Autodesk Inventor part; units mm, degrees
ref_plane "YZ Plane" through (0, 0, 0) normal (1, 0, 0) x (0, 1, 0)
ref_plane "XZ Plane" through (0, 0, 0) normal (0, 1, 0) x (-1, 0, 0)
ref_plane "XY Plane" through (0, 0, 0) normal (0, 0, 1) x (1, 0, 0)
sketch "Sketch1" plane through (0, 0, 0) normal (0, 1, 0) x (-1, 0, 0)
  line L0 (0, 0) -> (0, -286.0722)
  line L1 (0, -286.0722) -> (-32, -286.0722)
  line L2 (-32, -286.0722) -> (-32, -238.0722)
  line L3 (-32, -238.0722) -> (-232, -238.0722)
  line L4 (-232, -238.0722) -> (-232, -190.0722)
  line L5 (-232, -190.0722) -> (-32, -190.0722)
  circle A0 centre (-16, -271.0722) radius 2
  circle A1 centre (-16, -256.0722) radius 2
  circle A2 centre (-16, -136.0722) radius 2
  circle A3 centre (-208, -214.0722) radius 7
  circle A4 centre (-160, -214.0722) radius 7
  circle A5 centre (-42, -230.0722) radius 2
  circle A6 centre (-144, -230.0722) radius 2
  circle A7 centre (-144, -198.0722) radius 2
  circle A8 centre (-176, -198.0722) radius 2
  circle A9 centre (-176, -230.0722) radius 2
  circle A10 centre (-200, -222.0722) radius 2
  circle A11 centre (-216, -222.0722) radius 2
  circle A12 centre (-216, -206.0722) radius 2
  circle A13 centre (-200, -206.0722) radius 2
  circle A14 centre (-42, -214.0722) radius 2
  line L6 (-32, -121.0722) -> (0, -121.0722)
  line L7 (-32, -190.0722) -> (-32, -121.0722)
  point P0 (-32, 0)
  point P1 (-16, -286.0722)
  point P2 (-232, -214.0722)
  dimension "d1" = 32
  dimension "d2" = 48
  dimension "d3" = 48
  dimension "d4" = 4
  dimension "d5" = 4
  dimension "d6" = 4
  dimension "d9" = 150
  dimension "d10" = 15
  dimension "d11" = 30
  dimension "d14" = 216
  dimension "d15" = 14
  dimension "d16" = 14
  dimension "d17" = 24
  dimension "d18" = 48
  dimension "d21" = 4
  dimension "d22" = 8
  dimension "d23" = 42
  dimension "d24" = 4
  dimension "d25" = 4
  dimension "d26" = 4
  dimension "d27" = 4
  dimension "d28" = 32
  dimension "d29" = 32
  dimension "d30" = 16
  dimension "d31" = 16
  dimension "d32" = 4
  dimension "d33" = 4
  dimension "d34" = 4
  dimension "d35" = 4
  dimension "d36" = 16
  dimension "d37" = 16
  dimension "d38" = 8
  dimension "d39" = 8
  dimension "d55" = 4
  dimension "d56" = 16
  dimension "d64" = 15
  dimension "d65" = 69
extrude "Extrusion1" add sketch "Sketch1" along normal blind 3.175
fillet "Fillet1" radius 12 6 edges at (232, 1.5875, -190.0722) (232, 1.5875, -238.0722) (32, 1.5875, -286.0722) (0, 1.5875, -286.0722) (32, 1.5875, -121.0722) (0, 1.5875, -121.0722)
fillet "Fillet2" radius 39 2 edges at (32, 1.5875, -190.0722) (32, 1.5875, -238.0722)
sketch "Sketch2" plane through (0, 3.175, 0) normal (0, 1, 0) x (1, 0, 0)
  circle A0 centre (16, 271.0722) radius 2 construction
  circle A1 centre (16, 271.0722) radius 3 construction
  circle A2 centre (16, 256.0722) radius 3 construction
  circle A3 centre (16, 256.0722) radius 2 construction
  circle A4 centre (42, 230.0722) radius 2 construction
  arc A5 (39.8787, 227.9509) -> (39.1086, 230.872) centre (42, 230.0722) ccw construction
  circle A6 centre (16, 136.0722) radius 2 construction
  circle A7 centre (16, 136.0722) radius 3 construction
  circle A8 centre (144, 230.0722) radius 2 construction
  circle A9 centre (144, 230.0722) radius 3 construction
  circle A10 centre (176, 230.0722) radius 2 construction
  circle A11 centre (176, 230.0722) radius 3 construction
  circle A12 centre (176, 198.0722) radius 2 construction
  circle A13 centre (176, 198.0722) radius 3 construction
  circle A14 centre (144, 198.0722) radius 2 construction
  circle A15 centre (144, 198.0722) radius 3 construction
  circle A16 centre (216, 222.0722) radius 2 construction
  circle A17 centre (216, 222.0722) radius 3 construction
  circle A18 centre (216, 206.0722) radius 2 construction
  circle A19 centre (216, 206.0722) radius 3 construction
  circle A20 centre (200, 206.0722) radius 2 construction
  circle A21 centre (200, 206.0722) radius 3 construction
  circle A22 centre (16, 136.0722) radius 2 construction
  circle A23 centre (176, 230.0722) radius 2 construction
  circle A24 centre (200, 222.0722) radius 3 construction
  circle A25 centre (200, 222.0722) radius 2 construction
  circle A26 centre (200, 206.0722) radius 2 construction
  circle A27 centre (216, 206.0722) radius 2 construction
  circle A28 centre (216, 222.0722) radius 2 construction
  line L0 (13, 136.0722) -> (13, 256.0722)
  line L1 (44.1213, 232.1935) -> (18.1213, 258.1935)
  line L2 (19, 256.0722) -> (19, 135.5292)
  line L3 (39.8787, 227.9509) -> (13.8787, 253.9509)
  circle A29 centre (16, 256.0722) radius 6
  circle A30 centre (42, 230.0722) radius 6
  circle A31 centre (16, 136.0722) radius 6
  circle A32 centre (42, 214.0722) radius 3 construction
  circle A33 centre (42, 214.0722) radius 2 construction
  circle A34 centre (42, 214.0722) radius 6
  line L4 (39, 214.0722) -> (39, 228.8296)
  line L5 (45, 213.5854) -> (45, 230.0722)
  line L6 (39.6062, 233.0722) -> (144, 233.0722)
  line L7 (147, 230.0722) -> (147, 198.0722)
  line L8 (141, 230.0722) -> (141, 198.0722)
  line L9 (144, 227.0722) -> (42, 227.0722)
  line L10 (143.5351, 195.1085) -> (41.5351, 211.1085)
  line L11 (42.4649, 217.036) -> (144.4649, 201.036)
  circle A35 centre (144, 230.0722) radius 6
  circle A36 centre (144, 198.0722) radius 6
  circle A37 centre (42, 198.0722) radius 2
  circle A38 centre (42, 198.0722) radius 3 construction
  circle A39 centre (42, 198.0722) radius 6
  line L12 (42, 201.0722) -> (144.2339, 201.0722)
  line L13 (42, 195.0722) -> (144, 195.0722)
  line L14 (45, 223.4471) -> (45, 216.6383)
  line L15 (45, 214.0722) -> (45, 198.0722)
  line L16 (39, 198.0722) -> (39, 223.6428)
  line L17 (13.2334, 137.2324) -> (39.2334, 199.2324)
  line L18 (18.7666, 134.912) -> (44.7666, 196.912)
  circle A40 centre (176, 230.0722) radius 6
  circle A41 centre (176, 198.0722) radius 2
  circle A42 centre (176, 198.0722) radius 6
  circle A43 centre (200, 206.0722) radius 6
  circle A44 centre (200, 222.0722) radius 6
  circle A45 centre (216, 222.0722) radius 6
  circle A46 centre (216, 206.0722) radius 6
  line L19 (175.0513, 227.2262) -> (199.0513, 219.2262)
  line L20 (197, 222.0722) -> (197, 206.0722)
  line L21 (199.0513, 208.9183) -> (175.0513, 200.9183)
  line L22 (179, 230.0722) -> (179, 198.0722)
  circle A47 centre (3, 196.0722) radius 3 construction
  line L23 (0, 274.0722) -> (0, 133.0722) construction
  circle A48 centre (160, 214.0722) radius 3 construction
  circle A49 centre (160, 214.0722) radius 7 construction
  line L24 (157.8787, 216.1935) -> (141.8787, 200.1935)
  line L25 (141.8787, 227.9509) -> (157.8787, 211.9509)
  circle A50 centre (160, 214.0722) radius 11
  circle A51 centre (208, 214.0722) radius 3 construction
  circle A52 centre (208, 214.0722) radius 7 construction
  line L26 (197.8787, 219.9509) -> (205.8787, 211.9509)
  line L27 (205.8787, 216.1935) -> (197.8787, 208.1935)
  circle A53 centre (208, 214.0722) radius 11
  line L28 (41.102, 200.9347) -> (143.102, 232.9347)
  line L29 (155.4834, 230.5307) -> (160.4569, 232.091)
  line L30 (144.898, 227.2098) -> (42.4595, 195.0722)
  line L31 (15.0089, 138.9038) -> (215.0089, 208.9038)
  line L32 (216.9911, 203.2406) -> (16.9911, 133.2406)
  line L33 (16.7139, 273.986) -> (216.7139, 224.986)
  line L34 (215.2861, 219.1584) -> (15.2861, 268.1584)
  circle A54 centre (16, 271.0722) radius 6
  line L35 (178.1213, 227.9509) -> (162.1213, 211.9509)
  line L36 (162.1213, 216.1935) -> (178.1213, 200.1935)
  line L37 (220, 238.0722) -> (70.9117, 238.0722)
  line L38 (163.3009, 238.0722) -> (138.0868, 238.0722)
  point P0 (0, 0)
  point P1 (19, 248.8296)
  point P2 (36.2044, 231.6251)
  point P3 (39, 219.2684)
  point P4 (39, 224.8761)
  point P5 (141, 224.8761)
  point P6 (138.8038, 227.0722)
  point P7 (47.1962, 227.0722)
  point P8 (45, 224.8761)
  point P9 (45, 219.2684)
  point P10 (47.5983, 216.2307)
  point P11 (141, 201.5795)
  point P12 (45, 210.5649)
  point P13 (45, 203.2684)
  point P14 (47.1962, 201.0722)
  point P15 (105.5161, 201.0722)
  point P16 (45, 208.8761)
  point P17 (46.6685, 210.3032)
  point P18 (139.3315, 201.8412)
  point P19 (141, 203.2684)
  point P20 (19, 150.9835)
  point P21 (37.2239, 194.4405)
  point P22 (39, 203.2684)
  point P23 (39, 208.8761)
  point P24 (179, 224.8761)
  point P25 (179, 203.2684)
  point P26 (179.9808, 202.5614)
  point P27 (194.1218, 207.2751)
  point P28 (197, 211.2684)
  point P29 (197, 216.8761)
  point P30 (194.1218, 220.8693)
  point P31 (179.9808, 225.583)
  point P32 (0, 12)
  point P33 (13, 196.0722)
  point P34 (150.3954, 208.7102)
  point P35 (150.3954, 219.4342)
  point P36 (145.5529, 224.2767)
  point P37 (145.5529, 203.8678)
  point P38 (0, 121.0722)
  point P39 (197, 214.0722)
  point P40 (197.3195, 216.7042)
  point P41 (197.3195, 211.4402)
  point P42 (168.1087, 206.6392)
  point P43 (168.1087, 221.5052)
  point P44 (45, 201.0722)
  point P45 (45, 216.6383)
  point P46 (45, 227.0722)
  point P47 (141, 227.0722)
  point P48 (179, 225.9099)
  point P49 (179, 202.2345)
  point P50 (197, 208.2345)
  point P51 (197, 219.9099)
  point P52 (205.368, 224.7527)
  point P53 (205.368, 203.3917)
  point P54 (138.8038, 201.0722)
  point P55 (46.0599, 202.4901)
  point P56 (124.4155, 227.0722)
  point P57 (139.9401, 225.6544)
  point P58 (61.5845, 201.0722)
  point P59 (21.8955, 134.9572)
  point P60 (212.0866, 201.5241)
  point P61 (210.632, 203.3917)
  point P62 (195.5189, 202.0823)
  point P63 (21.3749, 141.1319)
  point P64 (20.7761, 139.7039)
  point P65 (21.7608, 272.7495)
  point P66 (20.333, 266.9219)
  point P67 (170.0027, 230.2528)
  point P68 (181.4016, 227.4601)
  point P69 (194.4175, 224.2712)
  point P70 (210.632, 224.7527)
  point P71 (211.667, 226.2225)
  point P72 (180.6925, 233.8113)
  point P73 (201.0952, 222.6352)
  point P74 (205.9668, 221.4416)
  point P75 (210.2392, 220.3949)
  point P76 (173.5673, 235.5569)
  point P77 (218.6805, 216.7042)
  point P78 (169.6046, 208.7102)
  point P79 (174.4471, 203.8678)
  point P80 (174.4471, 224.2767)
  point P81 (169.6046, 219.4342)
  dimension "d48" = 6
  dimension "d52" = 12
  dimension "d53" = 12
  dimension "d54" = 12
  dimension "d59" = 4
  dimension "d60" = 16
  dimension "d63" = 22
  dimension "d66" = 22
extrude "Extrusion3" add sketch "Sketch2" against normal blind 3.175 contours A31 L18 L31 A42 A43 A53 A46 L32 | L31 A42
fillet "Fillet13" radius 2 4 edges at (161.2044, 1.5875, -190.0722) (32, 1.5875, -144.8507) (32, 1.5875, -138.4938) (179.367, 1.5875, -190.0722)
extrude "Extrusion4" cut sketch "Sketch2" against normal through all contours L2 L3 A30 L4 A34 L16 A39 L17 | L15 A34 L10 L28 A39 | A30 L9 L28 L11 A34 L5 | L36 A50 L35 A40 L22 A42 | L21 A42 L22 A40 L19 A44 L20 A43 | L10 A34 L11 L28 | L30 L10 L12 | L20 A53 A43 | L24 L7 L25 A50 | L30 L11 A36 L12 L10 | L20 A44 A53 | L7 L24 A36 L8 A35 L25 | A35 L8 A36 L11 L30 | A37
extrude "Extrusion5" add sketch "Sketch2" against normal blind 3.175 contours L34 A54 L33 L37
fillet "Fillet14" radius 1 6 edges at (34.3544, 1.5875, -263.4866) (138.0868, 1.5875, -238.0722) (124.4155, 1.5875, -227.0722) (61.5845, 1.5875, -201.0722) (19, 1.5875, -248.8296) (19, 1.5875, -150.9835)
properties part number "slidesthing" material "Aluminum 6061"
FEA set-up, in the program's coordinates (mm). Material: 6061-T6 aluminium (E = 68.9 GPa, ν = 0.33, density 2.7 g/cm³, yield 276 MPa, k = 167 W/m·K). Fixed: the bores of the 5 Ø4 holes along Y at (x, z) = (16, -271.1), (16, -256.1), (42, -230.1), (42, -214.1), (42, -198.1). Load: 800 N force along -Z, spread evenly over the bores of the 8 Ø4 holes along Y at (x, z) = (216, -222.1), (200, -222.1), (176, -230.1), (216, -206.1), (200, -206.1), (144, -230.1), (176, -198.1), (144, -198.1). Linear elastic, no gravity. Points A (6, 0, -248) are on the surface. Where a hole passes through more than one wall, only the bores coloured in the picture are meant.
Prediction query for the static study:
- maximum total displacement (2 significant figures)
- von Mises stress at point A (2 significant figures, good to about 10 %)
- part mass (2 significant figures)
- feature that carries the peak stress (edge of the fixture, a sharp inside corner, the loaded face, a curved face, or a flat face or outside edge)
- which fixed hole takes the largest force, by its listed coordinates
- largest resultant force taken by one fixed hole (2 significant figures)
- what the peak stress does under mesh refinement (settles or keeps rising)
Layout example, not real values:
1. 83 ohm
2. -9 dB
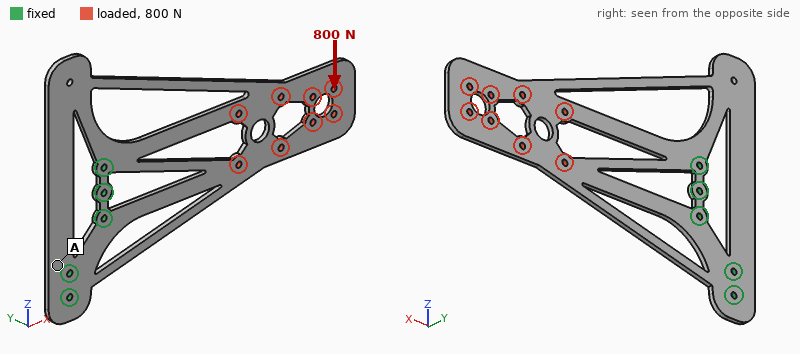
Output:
1. 0.41 mm
2. 14 MPa
3. 110 g
4. edge of the fixture
5. (42, -198.1)
6. 1.9 kN
7. keeps rising
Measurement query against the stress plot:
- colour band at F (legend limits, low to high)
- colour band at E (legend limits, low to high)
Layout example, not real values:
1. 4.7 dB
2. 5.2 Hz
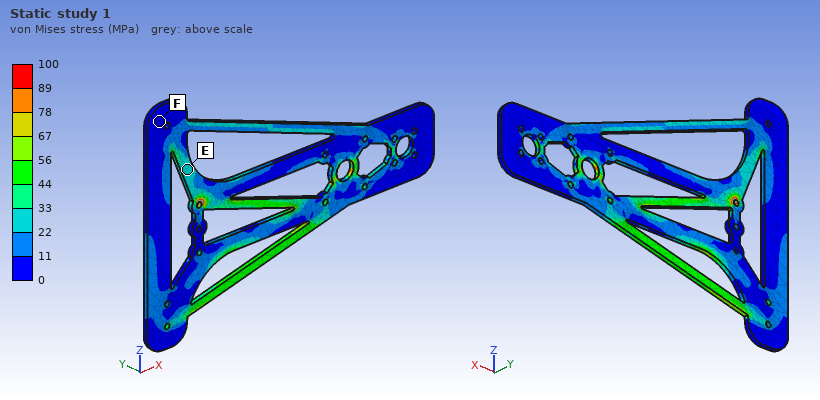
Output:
1. 0 to 11 MPa
2. 22 to 33 MPa
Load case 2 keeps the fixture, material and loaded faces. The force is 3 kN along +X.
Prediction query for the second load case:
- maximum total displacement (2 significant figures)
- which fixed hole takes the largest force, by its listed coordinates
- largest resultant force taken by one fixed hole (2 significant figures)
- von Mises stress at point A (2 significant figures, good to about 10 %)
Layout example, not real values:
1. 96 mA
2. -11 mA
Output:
1. 74 µm
2. (42, -198.1)
3. 1.7 kN
4. 6.0 MPa
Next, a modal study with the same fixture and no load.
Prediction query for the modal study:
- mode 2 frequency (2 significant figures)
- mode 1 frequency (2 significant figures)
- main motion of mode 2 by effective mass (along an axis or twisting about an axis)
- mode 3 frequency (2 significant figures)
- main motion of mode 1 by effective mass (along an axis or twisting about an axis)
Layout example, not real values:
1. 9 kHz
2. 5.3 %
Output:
1. 310 Hz
2. 71 Hz
3. along Y
4. 390 Hz
5. along Y
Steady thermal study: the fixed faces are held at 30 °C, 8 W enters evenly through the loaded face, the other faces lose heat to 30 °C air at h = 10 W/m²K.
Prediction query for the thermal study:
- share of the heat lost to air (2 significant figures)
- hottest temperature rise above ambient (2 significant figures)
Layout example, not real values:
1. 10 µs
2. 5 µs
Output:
1. 50 %
2. 36 K
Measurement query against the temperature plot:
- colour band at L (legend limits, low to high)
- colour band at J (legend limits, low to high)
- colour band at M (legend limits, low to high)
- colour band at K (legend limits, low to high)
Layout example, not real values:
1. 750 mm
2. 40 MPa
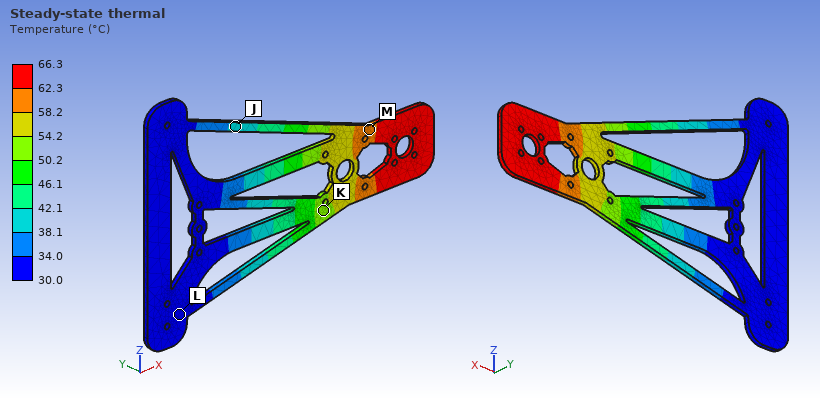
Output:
1. 30.0 to 34.0 °C
2. 38.1 to 42.1 °C
3. 58.2 to 62.3 °C
4. 50.2 to 54.2 °C
